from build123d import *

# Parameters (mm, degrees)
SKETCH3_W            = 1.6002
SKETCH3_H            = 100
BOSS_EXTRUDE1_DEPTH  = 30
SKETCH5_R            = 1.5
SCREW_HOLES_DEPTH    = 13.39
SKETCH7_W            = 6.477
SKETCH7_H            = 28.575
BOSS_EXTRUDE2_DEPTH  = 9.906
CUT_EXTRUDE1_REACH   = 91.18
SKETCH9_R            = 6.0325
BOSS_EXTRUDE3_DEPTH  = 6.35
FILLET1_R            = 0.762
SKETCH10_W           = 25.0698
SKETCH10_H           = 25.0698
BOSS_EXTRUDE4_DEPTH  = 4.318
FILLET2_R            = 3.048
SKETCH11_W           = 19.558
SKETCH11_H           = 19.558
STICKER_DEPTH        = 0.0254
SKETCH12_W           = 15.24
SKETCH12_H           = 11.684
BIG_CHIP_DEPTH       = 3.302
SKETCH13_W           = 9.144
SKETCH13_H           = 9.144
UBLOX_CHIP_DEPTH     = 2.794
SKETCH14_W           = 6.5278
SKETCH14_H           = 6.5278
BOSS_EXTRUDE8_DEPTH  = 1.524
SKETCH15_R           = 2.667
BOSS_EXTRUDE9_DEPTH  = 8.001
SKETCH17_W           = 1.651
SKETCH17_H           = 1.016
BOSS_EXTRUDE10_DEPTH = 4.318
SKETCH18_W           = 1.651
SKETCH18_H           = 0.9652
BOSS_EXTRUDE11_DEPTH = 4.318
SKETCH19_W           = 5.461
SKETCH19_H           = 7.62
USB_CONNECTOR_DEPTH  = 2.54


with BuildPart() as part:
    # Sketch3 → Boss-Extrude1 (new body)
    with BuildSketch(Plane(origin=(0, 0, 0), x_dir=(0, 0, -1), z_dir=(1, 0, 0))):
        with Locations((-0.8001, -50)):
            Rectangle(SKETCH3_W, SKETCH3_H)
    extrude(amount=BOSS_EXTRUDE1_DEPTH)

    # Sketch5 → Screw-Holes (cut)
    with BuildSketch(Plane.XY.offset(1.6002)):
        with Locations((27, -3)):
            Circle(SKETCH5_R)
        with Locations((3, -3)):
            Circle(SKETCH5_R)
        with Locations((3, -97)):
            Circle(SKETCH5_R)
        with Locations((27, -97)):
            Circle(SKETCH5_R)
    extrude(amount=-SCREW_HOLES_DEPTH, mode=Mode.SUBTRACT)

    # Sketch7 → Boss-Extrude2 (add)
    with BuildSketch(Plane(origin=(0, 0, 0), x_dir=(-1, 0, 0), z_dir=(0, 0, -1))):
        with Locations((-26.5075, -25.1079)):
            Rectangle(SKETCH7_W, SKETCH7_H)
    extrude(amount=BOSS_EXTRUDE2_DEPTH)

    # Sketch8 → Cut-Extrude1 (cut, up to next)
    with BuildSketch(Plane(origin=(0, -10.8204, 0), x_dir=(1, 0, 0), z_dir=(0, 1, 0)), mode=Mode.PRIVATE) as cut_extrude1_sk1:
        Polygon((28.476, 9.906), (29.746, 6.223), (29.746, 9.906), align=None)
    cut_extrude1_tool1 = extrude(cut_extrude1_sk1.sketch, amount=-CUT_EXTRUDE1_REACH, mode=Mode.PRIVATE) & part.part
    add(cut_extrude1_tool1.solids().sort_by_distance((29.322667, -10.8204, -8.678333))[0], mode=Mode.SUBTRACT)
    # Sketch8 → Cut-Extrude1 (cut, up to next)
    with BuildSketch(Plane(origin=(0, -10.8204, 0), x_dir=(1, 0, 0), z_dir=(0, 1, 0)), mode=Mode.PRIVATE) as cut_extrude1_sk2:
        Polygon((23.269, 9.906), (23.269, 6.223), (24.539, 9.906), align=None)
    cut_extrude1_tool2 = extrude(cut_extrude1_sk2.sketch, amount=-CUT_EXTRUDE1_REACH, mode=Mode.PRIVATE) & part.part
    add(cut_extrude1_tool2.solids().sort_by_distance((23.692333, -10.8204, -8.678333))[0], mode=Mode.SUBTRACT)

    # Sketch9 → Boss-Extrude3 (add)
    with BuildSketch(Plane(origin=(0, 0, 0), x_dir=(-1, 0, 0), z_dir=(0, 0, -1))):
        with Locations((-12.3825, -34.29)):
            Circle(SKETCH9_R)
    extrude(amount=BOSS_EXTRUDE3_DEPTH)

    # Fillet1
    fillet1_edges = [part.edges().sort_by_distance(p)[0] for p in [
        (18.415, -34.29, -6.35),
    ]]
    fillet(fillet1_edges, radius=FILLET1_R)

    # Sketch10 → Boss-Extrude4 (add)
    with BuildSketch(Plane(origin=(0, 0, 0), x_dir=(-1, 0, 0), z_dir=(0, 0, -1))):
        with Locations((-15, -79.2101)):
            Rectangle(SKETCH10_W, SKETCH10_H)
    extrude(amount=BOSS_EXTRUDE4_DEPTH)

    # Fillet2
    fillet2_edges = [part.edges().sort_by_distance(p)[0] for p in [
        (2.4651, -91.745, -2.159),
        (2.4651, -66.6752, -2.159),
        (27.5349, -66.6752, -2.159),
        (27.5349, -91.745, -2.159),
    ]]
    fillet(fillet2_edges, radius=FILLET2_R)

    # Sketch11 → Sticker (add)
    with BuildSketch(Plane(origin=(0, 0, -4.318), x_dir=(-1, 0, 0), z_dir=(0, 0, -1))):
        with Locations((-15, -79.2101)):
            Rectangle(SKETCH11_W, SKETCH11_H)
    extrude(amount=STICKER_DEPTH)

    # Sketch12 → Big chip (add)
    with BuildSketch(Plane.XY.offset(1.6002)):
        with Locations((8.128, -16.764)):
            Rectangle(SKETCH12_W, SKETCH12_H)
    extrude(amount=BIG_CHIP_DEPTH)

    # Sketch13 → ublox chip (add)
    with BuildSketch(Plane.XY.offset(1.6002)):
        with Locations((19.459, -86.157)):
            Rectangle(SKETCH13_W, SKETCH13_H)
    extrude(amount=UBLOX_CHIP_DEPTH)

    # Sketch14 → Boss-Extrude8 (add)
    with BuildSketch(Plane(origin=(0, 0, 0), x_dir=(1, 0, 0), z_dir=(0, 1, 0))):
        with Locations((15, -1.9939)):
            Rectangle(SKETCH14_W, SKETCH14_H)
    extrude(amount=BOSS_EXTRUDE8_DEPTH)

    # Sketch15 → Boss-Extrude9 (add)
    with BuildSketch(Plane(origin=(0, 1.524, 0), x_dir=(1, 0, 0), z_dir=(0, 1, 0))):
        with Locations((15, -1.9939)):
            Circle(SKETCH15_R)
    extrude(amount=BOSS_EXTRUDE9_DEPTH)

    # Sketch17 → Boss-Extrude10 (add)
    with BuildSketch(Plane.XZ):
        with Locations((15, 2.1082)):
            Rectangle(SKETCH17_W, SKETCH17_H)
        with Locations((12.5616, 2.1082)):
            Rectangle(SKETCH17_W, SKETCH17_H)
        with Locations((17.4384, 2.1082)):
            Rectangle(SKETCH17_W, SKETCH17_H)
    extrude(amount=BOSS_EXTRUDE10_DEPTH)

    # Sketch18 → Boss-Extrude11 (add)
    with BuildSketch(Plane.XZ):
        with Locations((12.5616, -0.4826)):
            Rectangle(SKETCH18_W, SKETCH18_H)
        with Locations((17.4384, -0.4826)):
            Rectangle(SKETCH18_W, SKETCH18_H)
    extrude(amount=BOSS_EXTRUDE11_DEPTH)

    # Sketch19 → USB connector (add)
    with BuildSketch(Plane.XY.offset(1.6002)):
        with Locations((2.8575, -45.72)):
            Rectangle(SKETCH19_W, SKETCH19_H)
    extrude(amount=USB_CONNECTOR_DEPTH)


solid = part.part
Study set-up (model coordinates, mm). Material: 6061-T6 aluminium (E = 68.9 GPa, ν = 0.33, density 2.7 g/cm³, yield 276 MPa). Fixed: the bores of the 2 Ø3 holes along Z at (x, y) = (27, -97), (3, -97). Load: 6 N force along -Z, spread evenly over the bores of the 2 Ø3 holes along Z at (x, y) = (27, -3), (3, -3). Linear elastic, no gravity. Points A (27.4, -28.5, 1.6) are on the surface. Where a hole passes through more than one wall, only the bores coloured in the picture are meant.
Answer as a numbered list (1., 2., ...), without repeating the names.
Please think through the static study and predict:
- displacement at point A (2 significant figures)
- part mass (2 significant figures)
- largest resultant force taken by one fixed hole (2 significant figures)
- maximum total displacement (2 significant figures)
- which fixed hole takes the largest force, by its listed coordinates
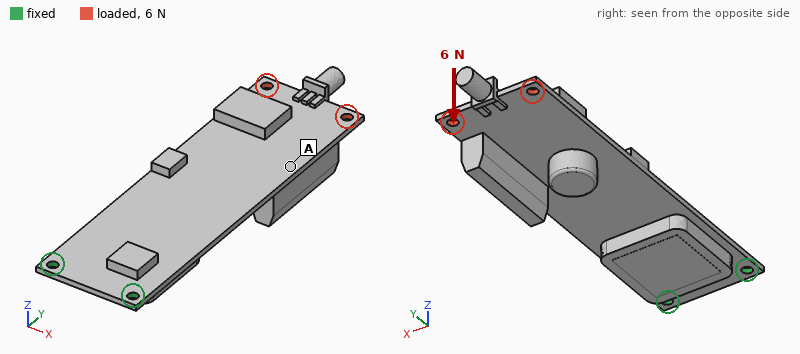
1. 0.63 mm
2. 30 g
3. 3.2 N
4. 1.3 mm
5. (3, -97)
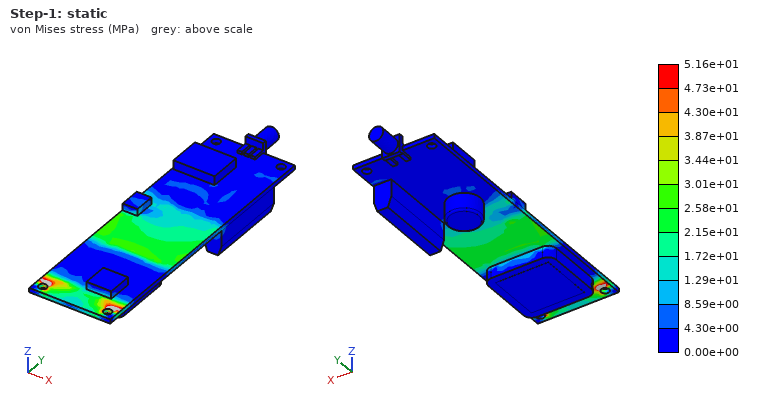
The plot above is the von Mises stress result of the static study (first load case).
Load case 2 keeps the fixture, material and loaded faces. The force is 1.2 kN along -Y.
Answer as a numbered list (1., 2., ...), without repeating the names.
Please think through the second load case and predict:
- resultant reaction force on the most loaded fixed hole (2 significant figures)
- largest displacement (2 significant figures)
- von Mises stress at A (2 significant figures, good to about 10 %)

1. 620 N
2. 0.18 mm
3. 16 MPa
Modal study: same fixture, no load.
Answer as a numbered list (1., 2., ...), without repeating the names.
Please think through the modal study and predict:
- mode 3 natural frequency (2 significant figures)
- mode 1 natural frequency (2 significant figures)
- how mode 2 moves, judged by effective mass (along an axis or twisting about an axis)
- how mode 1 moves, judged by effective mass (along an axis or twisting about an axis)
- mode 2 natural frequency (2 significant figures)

1. 980 Hz
2. 140 Hz
3. along Z
4. along Z
5. 790 Hz
